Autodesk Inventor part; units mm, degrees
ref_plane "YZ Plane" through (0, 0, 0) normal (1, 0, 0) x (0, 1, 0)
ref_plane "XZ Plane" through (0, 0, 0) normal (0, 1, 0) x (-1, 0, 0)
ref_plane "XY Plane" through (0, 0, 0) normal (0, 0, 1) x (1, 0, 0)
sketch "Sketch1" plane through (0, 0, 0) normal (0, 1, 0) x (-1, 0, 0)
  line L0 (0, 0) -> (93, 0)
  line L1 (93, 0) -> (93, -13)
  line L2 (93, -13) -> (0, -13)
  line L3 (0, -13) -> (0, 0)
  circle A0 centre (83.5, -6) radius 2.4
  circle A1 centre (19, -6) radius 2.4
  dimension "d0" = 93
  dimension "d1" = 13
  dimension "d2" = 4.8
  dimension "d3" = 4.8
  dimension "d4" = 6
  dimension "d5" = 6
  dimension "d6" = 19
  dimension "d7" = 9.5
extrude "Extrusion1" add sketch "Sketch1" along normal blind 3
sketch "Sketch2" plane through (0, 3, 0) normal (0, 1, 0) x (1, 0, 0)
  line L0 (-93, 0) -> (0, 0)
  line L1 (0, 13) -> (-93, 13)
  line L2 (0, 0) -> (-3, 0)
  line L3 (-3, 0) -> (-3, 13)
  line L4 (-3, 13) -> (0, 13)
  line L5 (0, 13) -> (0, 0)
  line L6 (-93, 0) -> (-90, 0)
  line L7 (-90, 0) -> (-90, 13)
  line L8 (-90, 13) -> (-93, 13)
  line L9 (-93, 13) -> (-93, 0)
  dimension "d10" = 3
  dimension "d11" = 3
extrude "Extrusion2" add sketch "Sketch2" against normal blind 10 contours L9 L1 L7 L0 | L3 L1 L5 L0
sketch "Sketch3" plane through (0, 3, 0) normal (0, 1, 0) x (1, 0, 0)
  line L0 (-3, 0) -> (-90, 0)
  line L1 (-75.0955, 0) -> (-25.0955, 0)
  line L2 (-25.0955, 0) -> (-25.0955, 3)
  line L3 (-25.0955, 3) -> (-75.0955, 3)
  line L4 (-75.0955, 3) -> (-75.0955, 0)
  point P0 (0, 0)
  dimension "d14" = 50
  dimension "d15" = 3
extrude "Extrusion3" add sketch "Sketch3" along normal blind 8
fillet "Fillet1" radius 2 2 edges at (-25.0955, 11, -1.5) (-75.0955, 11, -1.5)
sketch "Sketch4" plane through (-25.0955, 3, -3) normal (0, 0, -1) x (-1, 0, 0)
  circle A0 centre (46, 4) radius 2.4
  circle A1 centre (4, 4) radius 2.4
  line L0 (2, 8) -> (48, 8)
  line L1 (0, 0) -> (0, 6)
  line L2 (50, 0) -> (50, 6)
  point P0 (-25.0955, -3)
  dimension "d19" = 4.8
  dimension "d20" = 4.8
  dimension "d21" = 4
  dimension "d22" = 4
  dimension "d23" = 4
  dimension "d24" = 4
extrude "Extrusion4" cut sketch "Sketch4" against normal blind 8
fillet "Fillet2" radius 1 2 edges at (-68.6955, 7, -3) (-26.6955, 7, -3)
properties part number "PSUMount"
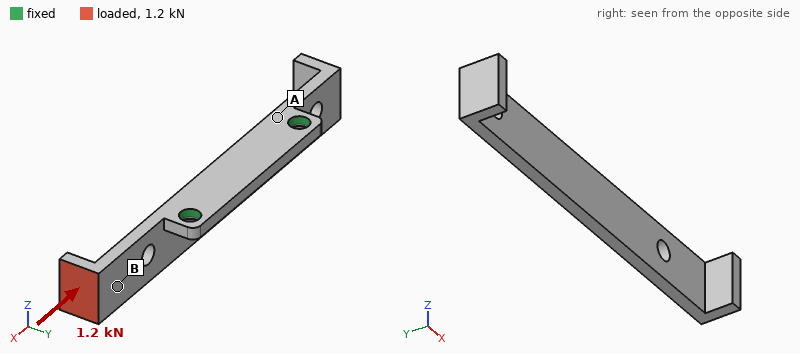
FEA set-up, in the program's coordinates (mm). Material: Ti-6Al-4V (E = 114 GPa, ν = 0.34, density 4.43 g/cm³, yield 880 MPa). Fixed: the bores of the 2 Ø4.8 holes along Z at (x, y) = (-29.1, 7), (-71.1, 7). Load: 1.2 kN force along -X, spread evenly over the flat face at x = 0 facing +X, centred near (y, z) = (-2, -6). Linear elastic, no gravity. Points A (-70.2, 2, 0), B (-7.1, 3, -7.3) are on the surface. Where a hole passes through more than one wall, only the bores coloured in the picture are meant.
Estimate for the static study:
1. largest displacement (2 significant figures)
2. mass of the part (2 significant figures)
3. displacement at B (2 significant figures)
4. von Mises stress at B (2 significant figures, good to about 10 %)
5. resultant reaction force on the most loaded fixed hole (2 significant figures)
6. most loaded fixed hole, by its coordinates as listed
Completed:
0.74 mm
23 g
0.38 mm
170 MPa
680 N
(-29.1, 7)
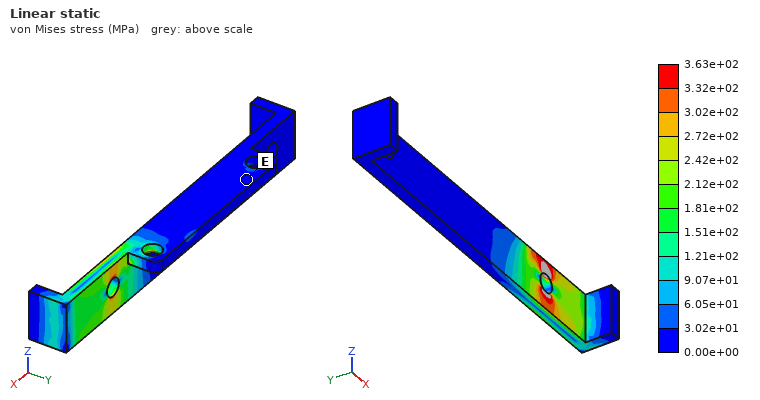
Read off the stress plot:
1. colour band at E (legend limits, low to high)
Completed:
0.00e+00 to 3.02e+01 MPa
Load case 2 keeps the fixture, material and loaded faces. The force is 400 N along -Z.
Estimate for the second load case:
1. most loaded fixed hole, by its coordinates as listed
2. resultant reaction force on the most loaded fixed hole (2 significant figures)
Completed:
(-29.1, 7)
780 N
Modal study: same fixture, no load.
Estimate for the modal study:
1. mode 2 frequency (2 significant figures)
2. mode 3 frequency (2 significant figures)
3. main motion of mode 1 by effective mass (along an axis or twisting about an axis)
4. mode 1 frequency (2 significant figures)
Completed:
3100 Hz
4600 Hz
along Y
1900 Hz
